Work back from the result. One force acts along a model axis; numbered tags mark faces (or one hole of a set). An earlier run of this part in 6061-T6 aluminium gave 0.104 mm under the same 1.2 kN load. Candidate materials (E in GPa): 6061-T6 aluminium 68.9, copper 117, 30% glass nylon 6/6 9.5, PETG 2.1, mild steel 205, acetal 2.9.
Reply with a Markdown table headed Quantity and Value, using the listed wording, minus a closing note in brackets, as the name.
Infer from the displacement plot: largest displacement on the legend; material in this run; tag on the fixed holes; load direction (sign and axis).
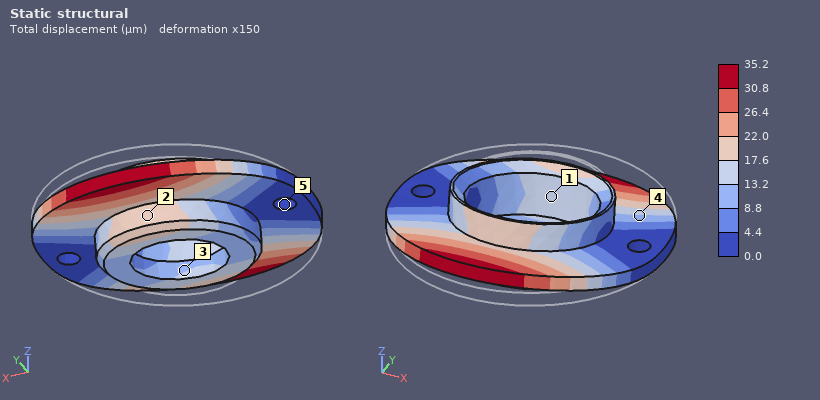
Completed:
| Quantity | Value |
|---|---|
| largest displacement on the legend | 35.2 µm |
| material in this run | mild steel |
| tag on the fixed holes | 5 |
| load direction | -Y |
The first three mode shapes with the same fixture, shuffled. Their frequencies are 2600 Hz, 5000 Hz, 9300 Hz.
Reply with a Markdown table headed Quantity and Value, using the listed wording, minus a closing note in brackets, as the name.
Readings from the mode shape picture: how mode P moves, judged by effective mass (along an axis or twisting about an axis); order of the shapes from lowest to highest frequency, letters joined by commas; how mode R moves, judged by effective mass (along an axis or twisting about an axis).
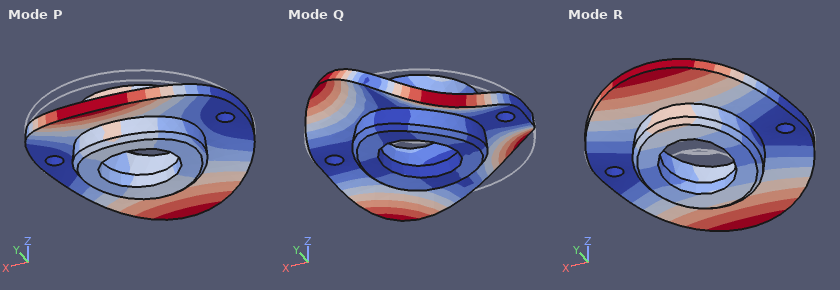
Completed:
| Quantity | Value |
|---|---|
| how mode P moves, judged by effective mass | along Z |
| order of the shapes from lowest to highest frequency, letters joined by commas | R, P, Q |
| how mode R moves, judged by effective mass | twisting about X |
